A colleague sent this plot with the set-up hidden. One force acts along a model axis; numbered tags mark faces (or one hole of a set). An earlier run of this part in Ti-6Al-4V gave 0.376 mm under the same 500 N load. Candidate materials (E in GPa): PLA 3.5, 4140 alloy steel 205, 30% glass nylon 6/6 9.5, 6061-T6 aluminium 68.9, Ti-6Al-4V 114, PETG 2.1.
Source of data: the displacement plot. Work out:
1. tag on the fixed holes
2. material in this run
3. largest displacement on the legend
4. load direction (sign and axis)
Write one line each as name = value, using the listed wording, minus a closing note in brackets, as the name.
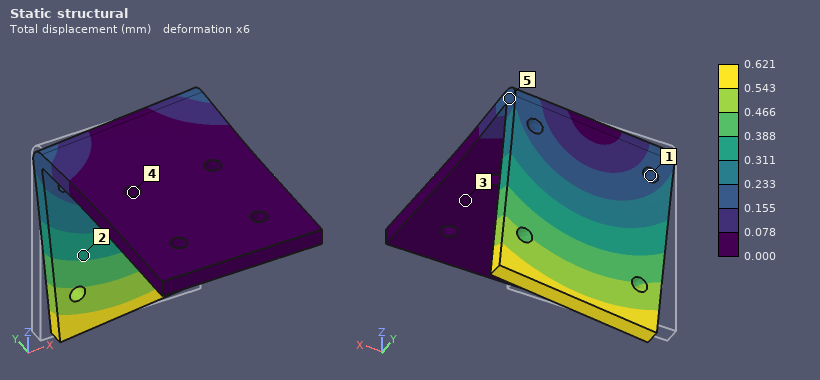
tag on the fixed holes = 4
material in this run = 6061-T6 aluminium
largest displacement on the legend = 0.621 mm
load direction = +X
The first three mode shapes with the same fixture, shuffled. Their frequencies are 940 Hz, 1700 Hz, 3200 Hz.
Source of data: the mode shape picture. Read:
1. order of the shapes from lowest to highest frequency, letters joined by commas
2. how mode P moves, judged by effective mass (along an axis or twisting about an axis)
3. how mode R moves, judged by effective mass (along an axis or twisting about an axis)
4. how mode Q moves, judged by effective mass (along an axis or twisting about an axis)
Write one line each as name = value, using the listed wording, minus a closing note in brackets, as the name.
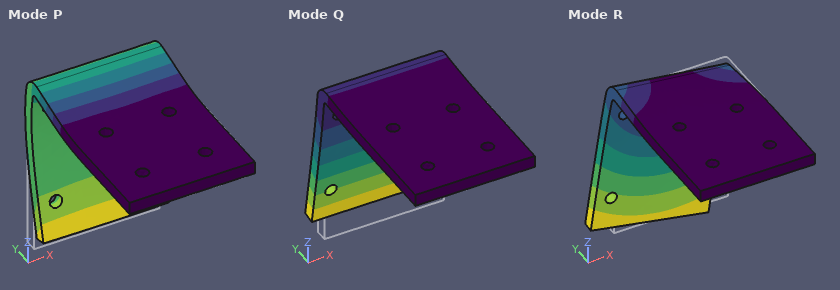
order of the shapes from lowest to highest frequency, letters joined by commas = Q, R, P
how mode P moves, judged by effective mass = along Z
how mode R moves, judged by effective mass = along X
how mode Q moves, judged by effective mass = along Y
